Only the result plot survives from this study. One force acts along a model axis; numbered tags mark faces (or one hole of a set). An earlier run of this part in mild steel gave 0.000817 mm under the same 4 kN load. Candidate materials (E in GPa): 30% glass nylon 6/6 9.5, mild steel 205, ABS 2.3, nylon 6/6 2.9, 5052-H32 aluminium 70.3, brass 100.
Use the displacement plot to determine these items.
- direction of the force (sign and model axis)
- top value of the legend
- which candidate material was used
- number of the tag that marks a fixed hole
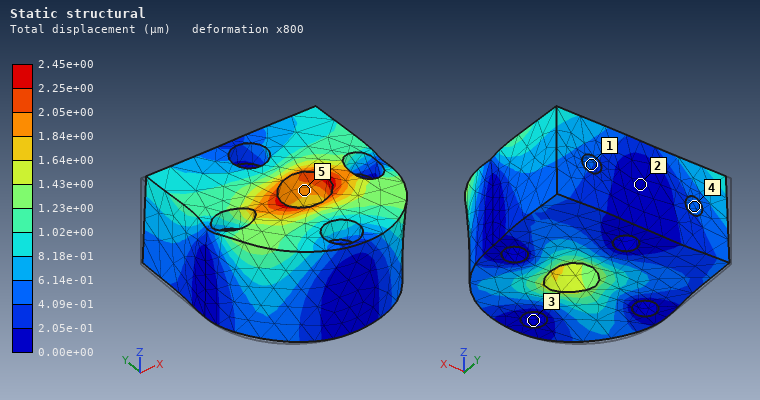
+X
2.45e+00 µm
5052-H32 aluminium
3
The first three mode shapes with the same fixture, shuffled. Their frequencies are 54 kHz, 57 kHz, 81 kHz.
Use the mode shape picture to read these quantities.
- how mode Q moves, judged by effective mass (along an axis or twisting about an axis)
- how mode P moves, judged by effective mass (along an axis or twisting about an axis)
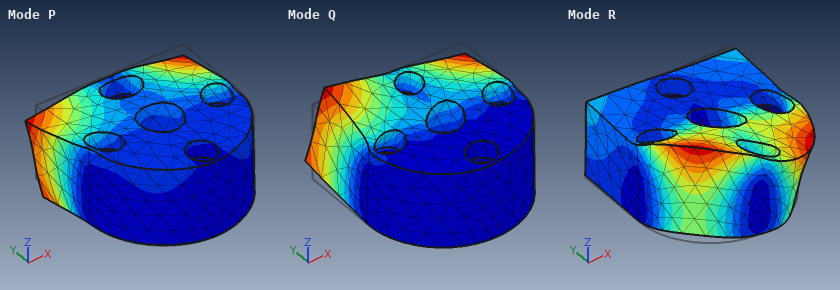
twisting about Y
along Z
